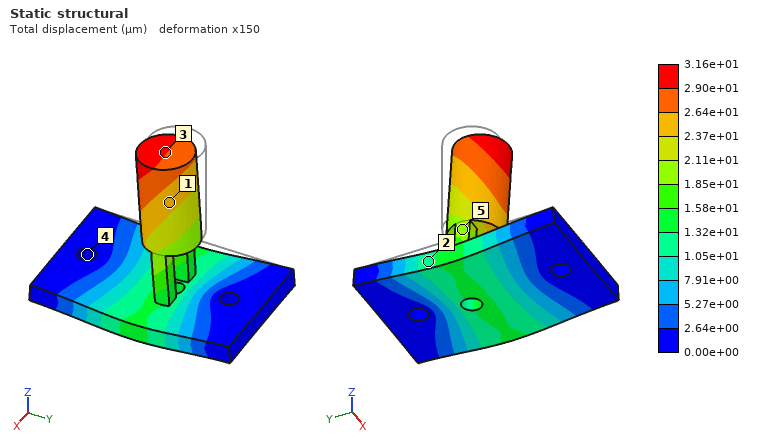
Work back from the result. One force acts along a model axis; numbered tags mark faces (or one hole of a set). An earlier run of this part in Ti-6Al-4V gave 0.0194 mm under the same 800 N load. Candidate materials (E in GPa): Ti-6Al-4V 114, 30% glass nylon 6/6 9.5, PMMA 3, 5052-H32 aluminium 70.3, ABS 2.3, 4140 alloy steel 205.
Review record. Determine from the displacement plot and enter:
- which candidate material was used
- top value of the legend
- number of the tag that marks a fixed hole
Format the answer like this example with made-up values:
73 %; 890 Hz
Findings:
5052-H32 aluminium; 3.16e+01 µm; 4
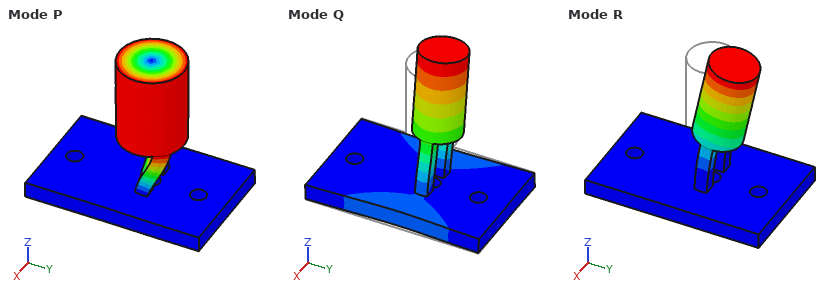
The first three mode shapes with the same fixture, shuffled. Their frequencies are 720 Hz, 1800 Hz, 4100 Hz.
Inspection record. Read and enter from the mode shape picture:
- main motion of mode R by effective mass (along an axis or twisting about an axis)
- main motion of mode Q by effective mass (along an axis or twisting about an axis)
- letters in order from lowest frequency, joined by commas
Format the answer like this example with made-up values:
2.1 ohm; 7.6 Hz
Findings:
along Y; along X; R, Q, P
